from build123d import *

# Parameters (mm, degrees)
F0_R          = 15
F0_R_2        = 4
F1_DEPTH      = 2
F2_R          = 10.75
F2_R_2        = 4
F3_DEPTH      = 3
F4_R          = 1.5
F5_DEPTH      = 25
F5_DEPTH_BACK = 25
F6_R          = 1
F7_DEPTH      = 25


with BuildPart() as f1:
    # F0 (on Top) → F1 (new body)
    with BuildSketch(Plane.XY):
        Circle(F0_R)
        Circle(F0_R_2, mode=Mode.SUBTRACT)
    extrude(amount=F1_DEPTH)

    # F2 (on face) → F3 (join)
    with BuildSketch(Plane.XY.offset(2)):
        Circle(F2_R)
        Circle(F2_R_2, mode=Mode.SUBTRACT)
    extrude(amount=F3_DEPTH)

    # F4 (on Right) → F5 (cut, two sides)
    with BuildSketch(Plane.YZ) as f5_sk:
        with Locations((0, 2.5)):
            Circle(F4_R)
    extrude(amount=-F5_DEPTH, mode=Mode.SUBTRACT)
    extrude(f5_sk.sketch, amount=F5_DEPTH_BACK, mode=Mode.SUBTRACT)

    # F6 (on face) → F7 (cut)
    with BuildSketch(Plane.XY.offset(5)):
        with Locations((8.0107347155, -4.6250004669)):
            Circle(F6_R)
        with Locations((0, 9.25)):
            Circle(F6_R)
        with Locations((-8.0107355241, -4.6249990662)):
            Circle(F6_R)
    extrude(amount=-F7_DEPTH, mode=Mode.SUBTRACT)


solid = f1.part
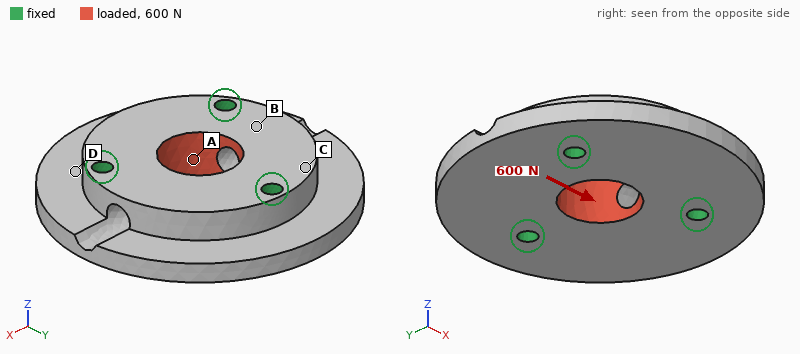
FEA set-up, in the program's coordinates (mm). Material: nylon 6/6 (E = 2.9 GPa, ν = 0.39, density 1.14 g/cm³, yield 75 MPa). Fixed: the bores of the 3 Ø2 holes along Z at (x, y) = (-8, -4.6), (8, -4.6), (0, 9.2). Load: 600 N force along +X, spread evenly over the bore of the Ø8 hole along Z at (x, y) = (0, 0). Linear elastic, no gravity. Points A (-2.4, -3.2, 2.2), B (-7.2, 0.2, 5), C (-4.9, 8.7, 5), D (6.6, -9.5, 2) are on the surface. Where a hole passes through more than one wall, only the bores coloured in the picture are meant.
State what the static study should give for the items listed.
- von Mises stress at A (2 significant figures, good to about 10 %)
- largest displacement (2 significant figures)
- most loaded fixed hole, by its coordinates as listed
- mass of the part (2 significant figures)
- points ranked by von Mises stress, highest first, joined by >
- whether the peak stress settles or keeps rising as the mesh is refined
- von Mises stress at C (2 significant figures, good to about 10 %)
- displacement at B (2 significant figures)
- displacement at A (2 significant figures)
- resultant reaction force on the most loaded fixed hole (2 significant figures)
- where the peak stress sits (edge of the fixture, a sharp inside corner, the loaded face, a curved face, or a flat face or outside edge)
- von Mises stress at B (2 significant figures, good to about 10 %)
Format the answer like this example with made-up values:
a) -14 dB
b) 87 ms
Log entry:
a) 8.6 MPa
b) 29 µm
c) (0, 9.2)
d) 2.4 g
e) A > B > C > D
f) keeps rising
g) 4.1 MPa
h) 19 µm
i) 14 µm
j) 220 N
k) edge of the fixture
l) 6.4 MPa
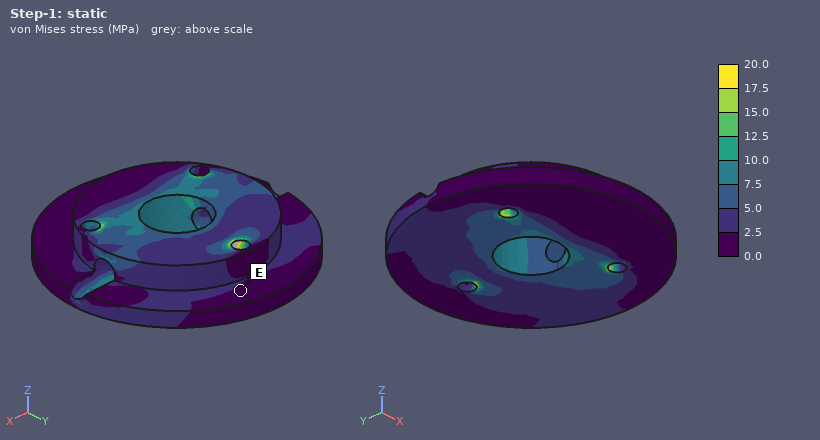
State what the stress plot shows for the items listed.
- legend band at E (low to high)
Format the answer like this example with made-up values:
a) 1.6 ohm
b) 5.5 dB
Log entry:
a) 0.0 to 2.5 MPa
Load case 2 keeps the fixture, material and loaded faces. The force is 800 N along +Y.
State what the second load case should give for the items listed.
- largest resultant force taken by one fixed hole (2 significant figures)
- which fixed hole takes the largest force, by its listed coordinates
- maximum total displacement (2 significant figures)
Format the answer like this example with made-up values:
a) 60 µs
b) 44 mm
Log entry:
a) 290 N
b) (0, 9.2)
c) 43 µm
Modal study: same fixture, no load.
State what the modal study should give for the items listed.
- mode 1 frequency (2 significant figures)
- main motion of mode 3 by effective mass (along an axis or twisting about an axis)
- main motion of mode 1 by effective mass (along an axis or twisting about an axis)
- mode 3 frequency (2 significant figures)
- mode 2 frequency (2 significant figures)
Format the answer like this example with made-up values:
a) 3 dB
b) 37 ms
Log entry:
a) 9300 Hz
b) along Z
c) twisting about Y
d) 11 kHz
e) 9800 Hz
